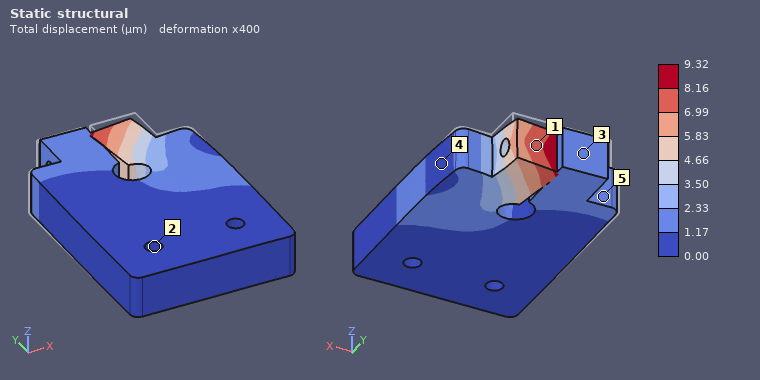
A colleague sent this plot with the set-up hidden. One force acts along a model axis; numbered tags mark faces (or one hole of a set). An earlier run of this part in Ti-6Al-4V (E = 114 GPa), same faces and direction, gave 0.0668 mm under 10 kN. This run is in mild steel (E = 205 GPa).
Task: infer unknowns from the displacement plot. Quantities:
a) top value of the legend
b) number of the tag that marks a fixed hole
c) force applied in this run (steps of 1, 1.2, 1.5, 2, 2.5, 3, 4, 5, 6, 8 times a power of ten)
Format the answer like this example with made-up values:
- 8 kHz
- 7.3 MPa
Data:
- 9.32 µm
- 2
- 2.5 kN
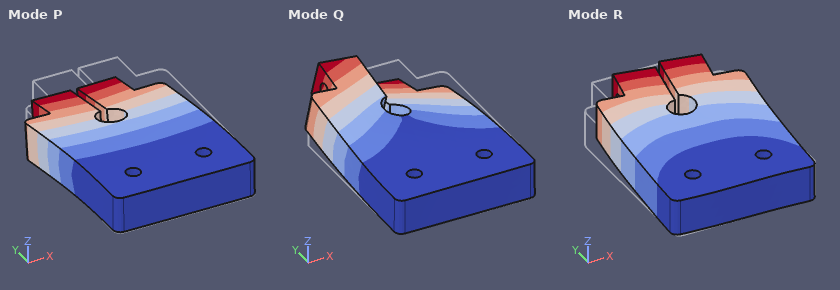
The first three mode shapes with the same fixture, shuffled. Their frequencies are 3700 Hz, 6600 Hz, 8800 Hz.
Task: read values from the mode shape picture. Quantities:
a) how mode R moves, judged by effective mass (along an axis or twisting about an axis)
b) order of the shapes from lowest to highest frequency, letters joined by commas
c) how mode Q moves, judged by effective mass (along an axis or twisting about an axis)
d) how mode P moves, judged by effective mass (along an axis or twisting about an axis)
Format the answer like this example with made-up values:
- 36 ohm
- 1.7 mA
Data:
- along X
- P, Q, R
- twisting about Y
- along Z
